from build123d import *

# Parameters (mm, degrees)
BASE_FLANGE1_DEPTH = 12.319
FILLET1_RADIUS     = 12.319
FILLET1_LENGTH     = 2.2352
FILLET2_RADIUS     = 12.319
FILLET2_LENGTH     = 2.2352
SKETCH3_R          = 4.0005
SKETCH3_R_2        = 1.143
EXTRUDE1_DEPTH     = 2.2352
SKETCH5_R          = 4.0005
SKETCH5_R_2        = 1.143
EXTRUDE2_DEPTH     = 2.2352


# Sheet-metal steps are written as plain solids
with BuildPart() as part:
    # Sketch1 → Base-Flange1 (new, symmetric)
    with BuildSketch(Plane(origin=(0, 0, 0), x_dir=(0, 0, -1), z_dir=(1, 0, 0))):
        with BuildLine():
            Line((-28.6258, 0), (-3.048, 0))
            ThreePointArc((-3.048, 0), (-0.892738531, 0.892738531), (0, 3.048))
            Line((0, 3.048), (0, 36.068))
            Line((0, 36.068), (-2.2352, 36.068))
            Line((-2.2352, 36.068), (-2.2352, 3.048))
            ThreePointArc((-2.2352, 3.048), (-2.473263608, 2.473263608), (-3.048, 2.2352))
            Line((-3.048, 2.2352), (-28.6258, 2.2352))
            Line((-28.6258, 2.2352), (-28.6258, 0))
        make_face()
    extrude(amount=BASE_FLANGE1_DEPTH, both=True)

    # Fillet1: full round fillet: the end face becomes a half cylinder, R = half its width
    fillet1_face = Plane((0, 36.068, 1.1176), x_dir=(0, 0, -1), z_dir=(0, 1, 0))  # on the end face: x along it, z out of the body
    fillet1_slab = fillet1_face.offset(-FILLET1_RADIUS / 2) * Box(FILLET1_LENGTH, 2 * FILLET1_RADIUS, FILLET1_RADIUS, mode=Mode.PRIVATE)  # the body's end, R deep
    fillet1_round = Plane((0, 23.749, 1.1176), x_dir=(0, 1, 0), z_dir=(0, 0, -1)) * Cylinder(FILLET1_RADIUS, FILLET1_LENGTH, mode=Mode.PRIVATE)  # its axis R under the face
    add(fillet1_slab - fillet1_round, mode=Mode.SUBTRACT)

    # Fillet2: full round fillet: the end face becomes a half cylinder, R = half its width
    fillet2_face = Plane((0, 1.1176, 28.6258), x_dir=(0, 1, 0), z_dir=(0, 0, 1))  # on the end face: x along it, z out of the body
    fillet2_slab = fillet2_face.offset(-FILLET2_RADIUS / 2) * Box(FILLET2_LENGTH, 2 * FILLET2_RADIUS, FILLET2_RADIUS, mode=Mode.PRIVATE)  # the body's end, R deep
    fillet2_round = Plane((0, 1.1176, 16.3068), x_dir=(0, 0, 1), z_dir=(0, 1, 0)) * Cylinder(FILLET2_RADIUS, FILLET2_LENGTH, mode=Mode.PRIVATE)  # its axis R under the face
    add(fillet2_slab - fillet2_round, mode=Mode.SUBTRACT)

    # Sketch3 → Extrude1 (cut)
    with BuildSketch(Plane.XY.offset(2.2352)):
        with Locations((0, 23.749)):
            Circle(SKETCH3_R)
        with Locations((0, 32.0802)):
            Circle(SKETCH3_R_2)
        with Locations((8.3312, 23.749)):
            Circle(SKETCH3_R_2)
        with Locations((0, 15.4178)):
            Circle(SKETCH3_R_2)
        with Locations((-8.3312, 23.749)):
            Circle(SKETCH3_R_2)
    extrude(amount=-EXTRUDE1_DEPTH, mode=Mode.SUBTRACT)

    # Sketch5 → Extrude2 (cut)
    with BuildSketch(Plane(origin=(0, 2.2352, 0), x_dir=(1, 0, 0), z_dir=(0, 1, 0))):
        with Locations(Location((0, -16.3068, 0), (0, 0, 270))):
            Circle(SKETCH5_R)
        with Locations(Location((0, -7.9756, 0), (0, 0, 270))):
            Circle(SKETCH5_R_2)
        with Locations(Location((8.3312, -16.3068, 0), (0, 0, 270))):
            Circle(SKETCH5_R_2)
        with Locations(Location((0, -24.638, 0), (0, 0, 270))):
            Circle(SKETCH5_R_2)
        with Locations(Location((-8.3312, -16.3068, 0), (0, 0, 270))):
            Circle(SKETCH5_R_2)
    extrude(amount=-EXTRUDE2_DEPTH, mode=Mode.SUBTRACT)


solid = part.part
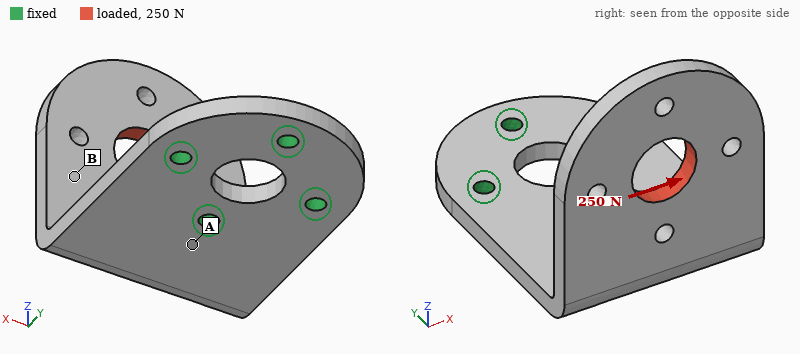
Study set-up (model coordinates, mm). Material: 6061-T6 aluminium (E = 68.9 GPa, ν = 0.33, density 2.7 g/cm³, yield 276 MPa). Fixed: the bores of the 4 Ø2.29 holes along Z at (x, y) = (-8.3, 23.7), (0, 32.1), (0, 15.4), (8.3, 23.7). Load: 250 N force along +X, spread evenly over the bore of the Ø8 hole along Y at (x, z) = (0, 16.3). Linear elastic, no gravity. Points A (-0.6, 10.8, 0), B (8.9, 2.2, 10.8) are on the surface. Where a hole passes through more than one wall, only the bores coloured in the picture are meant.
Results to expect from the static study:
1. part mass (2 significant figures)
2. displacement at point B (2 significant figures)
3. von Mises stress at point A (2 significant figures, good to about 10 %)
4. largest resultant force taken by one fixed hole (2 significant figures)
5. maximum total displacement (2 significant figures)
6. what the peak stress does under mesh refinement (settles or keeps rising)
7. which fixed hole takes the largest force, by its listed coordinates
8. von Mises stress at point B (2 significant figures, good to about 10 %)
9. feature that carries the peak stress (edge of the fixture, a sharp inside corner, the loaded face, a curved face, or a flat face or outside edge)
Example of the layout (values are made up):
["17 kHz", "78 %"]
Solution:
["7.6 g", "0.27 mm", "140 MPa", "280 N", "0.56 mm", "keeps rising", "(0, 15.4)", "35 MPa", "edge of the fixture"]
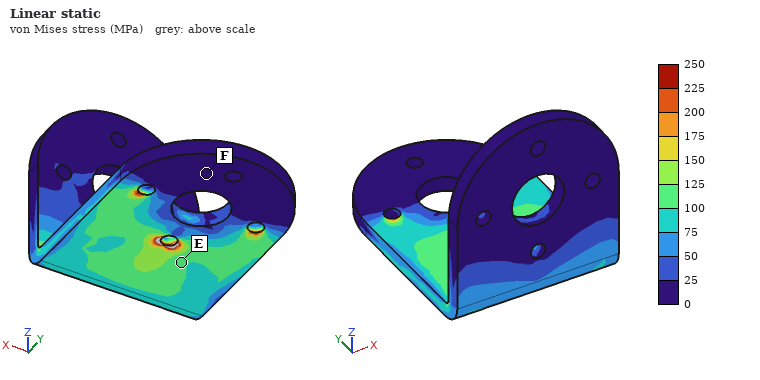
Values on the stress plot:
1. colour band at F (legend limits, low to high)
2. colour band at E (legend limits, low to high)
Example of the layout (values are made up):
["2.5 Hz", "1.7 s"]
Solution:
["0 to 25 MPa", "100 to 125 MPa"]
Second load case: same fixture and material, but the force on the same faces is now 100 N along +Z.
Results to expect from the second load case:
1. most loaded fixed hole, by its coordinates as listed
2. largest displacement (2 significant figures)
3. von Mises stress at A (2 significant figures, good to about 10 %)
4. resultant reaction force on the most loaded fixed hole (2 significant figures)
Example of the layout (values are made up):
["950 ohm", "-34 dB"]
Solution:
["(0, 15.4)", "0.21 mm", "55 MPa", "170 N"]
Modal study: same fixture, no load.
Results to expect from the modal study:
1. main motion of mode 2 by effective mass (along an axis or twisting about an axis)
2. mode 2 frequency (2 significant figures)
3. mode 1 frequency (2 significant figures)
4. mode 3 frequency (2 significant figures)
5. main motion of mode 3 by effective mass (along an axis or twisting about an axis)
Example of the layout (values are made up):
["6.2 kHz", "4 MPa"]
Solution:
["along X", "2300 Hz", "1600 Hz", "4500 Hz", "along Z"]
